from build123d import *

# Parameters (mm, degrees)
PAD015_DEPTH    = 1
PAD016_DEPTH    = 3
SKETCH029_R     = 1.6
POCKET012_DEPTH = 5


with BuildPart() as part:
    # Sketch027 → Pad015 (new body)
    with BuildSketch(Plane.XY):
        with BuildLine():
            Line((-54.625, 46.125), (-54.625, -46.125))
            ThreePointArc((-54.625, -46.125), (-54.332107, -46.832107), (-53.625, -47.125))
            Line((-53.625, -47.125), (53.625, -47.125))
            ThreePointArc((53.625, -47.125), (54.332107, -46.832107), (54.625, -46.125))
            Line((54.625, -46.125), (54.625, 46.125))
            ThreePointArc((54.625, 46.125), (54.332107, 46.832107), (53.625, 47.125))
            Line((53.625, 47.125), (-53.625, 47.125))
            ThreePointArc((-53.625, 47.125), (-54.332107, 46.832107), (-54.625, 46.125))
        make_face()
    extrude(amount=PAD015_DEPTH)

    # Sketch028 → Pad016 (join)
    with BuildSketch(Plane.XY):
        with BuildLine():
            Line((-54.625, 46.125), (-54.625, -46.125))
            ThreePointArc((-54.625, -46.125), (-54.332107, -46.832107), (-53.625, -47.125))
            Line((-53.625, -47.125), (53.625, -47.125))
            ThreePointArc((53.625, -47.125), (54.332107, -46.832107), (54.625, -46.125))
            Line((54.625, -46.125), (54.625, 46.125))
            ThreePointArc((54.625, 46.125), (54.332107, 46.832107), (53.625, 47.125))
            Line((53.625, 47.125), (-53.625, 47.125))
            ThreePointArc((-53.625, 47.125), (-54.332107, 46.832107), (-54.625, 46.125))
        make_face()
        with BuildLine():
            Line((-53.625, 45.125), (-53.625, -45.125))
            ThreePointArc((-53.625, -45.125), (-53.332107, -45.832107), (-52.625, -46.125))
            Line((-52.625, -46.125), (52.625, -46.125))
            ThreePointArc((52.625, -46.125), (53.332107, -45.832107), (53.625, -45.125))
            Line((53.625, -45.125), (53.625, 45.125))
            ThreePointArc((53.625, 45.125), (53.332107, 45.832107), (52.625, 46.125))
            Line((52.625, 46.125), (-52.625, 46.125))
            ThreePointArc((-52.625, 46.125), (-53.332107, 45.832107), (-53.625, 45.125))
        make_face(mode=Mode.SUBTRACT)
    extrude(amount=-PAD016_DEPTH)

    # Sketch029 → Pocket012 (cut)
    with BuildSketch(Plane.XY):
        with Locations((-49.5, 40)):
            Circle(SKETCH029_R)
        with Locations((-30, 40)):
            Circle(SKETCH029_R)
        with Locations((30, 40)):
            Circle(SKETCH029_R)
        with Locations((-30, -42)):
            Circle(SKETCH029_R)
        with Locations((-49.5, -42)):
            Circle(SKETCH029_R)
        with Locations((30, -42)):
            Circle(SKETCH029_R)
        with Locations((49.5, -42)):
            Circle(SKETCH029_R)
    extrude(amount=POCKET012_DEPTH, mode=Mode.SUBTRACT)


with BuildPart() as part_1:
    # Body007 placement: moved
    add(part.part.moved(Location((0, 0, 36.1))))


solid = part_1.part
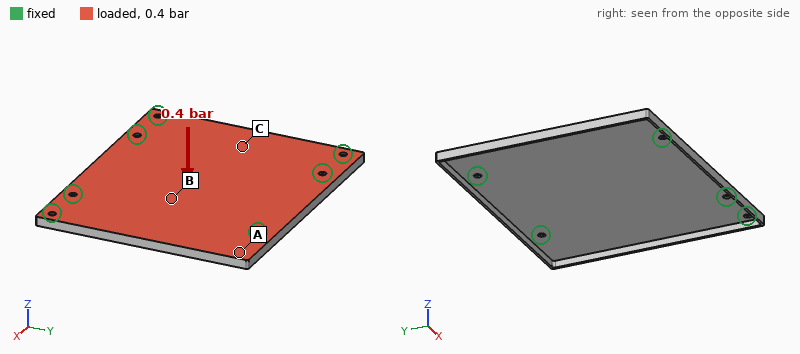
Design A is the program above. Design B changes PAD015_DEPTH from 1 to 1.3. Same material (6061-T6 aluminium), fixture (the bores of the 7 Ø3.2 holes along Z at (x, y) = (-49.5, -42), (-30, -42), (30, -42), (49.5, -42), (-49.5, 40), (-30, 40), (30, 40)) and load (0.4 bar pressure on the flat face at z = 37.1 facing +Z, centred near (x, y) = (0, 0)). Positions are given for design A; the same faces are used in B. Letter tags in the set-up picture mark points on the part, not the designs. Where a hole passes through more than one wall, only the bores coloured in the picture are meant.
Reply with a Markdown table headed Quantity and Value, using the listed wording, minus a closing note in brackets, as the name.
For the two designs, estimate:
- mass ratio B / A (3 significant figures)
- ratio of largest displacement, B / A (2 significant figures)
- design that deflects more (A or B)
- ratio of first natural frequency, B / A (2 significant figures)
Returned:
| Quantity | Value |
|---|---|
| mass ratio B / A | 1.27 |
| ratio of largest displacement, B / A | 0.47 |
| design that deflects more | A |
| ratio of first natural frequency, B / A | 1.3 |
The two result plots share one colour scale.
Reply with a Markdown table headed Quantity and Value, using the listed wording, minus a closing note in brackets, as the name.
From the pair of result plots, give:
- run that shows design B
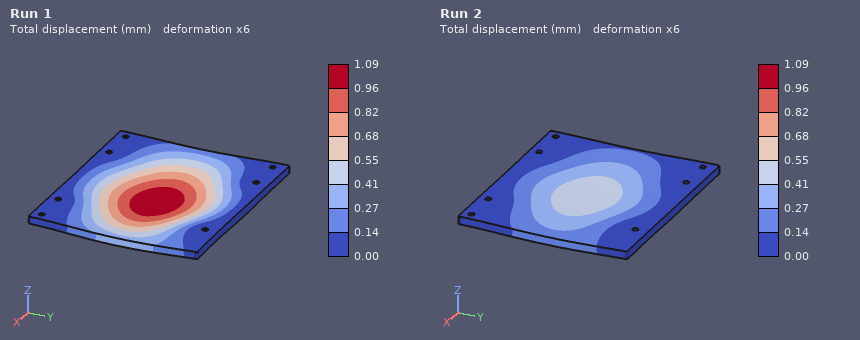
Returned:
| Quantity | Value |
|---|---|
| run that shows design B | Run 2 |
